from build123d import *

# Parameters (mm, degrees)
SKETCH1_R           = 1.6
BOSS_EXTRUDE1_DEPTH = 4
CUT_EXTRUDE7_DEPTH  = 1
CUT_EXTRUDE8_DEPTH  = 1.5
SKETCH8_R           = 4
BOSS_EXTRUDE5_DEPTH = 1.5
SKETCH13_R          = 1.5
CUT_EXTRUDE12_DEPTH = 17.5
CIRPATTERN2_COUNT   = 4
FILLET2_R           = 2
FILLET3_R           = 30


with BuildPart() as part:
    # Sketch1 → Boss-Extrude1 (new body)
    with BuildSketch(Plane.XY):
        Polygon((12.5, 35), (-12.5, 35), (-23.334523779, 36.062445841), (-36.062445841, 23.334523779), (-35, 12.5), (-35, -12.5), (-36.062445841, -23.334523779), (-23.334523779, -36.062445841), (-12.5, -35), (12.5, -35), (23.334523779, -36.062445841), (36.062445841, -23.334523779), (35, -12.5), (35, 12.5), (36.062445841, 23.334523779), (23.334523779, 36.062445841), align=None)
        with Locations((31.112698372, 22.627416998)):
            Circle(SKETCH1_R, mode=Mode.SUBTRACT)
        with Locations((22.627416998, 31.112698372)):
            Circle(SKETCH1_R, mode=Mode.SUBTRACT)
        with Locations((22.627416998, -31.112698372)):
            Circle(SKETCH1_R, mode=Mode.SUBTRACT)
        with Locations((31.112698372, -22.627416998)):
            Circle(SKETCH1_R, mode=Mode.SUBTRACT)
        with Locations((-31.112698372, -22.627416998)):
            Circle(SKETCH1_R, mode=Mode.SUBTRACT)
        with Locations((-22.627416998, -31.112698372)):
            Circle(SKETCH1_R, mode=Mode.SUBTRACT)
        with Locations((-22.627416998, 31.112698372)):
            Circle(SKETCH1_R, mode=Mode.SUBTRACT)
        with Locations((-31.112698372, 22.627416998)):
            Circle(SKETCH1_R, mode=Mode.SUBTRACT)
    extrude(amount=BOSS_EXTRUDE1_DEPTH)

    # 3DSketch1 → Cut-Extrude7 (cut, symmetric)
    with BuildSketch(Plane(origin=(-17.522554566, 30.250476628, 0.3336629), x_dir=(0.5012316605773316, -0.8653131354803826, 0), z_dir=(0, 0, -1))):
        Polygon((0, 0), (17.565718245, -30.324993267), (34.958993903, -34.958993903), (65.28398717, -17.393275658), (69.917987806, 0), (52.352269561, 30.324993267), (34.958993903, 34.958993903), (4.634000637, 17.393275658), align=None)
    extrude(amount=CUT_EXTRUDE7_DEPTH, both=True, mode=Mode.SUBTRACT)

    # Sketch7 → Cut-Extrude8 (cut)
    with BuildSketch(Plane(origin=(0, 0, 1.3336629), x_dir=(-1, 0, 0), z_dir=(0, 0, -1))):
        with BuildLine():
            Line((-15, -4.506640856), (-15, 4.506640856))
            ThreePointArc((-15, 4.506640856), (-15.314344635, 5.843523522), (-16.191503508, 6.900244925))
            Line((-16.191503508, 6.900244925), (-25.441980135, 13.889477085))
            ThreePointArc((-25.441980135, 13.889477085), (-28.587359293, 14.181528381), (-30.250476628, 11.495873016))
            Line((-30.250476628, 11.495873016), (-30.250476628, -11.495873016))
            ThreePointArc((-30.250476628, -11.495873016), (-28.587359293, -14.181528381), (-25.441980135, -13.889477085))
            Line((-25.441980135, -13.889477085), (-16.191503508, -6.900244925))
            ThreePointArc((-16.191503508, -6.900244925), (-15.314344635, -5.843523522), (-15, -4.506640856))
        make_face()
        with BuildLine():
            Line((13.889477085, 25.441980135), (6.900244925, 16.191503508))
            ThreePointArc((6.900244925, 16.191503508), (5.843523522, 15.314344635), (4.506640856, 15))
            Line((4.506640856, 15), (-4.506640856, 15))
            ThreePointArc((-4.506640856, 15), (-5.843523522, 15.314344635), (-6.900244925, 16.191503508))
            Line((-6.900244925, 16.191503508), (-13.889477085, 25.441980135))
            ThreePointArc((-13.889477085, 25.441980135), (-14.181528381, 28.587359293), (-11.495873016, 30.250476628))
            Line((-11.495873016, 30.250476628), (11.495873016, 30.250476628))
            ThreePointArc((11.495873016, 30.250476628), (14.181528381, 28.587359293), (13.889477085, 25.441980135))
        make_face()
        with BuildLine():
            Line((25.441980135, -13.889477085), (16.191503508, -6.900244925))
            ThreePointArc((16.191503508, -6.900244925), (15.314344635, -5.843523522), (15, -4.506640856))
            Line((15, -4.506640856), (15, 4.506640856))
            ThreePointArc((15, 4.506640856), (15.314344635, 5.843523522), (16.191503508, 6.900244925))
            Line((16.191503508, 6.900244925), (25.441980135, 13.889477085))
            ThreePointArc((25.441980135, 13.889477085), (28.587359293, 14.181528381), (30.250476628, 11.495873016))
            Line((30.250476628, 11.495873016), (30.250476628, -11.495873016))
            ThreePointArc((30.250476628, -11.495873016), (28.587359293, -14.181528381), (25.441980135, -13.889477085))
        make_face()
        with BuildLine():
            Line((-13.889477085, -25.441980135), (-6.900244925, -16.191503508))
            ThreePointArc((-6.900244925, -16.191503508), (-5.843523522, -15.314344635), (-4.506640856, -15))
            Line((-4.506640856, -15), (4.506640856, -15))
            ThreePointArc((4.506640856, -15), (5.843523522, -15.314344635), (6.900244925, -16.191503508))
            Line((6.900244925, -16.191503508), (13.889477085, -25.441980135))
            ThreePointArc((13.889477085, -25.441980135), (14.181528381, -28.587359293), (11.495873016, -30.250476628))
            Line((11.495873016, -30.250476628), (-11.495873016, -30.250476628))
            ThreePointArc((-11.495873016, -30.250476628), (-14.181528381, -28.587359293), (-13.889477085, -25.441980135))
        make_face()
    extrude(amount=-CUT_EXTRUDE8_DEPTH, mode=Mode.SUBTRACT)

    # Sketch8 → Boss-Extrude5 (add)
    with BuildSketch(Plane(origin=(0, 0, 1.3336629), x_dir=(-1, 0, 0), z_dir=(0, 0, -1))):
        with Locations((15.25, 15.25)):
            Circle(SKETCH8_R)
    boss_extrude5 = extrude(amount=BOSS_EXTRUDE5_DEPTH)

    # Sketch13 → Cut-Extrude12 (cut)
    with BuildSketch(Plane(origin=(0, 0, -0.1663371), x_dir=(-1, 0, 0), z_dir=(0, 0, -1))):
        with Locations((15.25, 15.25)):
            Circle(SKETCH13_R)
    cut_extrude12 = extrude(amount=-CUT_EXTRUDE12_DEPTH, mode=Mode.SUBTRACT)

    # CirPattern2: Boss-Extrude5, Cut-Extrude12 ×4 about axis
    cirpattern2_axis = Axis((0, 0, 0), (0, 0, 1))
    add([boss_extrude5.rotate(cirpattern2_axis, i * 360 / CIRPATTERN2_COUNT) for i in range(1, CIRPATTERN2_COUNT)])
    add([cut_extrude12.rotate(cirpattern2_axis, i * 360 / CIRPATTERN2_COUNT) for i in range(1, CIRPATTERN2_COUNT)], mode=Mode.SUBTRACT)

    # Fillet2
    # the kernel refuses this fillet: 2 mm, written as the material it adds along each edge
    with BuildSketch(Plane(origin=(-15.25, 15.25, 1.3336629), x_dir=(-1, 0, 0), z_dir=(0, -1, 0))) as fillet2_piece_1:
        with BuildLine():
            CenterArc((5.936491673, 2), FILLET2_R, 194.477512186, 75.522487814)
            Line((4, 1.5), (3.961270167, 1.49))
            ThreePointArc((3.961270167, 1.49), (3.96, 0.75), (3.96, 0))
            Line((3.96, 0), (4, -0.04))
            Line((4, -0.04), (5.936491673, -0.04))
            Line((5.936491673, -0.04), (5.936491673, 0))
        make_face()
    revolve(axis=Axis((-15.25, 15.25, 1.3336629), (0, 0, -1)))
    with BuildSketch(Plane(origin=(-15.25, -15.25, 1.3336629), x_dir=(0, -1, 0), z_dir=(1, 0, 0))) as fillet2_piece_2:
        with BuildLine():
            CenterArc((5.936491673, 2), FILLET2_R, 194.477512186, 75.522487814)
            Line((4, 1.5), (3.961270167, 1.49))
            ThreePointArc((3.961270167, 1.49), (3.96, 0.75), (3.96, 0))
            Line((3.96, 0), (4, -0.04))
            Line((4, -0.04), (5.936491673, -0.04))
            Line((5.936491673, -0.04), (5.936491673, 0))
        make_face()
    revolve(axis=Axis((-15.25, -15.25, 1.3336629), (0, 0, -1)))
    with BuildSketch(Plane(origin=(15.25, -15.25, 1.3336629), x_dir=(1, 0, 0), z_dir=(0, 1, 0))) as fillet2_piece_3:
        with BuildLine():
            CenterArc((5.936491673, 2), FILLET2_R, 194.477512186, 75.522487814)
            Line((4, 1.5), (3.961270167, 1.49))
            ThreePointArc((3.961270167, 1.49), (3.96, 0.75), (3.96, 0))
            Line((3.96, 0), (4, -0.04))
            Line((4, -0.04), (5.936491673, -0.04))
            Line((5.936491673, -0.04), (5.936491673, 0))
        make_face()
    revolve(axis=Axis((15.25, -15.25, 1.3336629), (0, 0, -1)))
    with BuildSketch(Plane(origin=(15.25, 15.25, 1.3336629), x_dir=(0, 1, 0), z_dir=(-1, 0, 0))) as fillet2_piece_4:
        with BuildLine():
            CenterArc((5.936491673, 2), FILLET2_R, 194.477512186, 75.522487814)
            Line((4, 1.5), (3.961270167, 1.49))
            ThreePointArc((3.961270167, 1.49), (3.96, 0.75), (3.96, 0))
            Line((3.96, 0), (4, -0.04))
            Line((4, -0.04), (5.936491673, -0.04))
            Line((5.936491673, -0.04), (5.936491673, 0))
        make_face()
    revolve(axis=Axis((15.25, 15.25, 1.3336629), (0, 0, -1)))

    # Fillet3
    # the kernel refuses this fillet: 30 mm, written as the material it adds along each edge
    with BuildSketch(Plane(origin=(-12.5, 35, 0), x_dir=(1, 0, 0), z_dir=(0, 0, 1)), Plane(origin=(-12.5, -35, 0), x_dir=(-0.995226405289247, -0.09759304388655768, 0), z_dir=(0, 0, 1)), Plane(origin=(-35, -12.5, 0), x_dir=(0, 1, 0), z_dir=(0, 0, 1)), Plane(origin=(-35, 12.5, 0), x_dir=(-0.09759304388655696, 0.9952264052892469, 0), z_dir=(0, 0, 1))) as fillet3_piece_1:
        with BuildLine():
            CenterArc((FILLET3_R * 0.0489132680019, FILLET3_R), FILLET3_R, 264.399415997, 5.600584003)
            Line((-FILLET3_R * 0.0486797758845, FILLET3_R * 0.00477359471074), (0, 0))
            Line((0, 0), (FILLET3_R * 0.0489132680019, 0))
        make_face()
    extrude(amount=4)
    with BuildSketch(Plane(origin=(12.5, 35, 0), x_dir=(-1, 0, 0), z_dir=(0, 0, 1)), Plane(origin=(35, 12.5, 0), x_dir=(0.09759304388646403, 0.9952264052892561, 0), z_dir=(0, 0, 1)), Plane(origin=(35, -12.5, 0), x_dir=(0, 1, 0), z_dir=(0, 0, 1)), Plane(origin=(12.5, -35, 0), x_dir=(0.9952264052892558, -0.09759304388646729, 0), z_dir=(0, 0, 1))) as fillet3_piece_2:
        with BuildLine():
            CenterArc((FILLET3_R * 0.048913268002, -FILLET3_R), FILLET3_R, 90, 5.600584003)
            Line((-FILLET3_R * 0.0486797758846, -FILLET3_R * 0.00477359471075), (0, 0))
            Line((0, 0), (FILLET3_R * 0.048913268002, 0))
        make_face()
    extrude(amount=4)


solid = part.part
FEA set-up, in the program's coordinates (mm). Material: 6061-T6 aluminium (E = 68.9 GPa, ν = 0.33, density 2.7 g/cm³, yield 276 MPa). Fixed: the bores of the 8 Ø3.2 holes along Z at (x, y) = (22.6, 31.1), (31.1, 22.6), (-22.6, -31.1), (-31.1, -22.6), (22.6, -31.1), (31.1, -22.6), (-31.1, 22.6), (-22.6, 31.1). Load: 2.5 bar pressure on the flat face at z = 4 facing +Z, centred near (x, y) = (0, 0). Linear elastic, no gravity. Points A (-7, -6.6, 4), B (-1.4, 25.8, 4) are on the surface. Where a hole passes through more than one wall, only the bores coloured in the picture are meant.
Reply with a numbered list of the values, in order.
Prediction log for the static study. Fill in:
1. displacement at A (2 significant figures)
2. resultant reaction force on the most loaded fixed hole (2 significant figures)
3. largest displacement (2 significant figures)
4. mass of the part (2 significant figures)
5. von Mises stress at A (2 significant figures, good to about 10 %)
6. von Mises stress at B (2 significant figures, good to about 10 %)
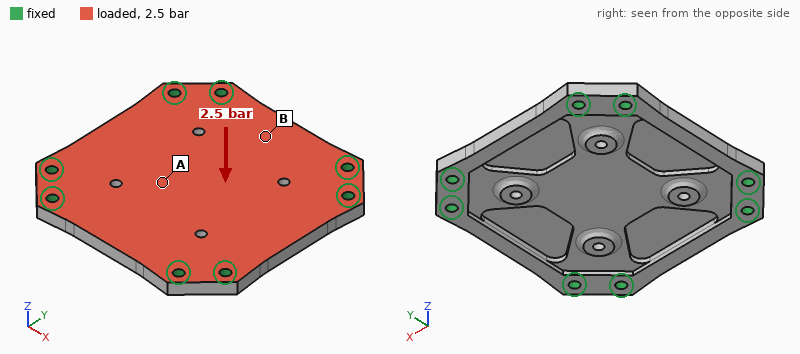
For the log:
1. 82 µm
2. 180 N
3. 92 µm
4. 34 g
5. 25 MPa
6. 17 MPa
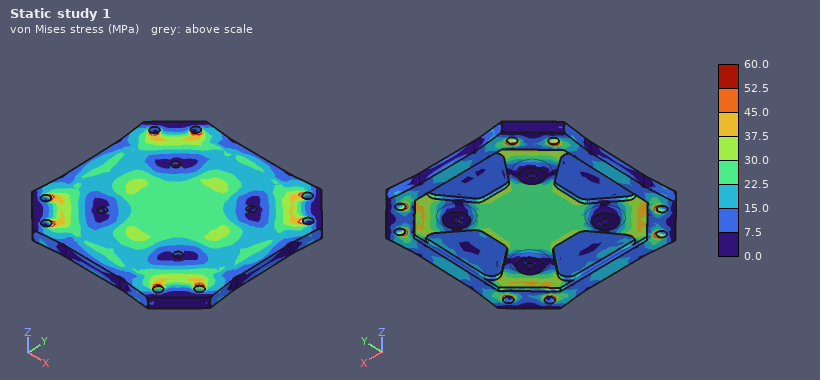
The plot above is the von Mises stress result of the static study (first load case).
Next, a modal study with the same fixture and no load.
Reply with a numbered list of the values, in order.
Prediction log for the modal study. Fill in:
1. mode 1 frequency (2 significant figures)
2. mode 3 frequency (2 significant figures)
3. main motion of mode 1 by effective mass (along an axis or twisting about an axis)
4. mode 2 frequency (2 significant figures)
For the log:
1. 4000 Hz
2. 8300 Hz
3. along Z
4. 8300 Hz
